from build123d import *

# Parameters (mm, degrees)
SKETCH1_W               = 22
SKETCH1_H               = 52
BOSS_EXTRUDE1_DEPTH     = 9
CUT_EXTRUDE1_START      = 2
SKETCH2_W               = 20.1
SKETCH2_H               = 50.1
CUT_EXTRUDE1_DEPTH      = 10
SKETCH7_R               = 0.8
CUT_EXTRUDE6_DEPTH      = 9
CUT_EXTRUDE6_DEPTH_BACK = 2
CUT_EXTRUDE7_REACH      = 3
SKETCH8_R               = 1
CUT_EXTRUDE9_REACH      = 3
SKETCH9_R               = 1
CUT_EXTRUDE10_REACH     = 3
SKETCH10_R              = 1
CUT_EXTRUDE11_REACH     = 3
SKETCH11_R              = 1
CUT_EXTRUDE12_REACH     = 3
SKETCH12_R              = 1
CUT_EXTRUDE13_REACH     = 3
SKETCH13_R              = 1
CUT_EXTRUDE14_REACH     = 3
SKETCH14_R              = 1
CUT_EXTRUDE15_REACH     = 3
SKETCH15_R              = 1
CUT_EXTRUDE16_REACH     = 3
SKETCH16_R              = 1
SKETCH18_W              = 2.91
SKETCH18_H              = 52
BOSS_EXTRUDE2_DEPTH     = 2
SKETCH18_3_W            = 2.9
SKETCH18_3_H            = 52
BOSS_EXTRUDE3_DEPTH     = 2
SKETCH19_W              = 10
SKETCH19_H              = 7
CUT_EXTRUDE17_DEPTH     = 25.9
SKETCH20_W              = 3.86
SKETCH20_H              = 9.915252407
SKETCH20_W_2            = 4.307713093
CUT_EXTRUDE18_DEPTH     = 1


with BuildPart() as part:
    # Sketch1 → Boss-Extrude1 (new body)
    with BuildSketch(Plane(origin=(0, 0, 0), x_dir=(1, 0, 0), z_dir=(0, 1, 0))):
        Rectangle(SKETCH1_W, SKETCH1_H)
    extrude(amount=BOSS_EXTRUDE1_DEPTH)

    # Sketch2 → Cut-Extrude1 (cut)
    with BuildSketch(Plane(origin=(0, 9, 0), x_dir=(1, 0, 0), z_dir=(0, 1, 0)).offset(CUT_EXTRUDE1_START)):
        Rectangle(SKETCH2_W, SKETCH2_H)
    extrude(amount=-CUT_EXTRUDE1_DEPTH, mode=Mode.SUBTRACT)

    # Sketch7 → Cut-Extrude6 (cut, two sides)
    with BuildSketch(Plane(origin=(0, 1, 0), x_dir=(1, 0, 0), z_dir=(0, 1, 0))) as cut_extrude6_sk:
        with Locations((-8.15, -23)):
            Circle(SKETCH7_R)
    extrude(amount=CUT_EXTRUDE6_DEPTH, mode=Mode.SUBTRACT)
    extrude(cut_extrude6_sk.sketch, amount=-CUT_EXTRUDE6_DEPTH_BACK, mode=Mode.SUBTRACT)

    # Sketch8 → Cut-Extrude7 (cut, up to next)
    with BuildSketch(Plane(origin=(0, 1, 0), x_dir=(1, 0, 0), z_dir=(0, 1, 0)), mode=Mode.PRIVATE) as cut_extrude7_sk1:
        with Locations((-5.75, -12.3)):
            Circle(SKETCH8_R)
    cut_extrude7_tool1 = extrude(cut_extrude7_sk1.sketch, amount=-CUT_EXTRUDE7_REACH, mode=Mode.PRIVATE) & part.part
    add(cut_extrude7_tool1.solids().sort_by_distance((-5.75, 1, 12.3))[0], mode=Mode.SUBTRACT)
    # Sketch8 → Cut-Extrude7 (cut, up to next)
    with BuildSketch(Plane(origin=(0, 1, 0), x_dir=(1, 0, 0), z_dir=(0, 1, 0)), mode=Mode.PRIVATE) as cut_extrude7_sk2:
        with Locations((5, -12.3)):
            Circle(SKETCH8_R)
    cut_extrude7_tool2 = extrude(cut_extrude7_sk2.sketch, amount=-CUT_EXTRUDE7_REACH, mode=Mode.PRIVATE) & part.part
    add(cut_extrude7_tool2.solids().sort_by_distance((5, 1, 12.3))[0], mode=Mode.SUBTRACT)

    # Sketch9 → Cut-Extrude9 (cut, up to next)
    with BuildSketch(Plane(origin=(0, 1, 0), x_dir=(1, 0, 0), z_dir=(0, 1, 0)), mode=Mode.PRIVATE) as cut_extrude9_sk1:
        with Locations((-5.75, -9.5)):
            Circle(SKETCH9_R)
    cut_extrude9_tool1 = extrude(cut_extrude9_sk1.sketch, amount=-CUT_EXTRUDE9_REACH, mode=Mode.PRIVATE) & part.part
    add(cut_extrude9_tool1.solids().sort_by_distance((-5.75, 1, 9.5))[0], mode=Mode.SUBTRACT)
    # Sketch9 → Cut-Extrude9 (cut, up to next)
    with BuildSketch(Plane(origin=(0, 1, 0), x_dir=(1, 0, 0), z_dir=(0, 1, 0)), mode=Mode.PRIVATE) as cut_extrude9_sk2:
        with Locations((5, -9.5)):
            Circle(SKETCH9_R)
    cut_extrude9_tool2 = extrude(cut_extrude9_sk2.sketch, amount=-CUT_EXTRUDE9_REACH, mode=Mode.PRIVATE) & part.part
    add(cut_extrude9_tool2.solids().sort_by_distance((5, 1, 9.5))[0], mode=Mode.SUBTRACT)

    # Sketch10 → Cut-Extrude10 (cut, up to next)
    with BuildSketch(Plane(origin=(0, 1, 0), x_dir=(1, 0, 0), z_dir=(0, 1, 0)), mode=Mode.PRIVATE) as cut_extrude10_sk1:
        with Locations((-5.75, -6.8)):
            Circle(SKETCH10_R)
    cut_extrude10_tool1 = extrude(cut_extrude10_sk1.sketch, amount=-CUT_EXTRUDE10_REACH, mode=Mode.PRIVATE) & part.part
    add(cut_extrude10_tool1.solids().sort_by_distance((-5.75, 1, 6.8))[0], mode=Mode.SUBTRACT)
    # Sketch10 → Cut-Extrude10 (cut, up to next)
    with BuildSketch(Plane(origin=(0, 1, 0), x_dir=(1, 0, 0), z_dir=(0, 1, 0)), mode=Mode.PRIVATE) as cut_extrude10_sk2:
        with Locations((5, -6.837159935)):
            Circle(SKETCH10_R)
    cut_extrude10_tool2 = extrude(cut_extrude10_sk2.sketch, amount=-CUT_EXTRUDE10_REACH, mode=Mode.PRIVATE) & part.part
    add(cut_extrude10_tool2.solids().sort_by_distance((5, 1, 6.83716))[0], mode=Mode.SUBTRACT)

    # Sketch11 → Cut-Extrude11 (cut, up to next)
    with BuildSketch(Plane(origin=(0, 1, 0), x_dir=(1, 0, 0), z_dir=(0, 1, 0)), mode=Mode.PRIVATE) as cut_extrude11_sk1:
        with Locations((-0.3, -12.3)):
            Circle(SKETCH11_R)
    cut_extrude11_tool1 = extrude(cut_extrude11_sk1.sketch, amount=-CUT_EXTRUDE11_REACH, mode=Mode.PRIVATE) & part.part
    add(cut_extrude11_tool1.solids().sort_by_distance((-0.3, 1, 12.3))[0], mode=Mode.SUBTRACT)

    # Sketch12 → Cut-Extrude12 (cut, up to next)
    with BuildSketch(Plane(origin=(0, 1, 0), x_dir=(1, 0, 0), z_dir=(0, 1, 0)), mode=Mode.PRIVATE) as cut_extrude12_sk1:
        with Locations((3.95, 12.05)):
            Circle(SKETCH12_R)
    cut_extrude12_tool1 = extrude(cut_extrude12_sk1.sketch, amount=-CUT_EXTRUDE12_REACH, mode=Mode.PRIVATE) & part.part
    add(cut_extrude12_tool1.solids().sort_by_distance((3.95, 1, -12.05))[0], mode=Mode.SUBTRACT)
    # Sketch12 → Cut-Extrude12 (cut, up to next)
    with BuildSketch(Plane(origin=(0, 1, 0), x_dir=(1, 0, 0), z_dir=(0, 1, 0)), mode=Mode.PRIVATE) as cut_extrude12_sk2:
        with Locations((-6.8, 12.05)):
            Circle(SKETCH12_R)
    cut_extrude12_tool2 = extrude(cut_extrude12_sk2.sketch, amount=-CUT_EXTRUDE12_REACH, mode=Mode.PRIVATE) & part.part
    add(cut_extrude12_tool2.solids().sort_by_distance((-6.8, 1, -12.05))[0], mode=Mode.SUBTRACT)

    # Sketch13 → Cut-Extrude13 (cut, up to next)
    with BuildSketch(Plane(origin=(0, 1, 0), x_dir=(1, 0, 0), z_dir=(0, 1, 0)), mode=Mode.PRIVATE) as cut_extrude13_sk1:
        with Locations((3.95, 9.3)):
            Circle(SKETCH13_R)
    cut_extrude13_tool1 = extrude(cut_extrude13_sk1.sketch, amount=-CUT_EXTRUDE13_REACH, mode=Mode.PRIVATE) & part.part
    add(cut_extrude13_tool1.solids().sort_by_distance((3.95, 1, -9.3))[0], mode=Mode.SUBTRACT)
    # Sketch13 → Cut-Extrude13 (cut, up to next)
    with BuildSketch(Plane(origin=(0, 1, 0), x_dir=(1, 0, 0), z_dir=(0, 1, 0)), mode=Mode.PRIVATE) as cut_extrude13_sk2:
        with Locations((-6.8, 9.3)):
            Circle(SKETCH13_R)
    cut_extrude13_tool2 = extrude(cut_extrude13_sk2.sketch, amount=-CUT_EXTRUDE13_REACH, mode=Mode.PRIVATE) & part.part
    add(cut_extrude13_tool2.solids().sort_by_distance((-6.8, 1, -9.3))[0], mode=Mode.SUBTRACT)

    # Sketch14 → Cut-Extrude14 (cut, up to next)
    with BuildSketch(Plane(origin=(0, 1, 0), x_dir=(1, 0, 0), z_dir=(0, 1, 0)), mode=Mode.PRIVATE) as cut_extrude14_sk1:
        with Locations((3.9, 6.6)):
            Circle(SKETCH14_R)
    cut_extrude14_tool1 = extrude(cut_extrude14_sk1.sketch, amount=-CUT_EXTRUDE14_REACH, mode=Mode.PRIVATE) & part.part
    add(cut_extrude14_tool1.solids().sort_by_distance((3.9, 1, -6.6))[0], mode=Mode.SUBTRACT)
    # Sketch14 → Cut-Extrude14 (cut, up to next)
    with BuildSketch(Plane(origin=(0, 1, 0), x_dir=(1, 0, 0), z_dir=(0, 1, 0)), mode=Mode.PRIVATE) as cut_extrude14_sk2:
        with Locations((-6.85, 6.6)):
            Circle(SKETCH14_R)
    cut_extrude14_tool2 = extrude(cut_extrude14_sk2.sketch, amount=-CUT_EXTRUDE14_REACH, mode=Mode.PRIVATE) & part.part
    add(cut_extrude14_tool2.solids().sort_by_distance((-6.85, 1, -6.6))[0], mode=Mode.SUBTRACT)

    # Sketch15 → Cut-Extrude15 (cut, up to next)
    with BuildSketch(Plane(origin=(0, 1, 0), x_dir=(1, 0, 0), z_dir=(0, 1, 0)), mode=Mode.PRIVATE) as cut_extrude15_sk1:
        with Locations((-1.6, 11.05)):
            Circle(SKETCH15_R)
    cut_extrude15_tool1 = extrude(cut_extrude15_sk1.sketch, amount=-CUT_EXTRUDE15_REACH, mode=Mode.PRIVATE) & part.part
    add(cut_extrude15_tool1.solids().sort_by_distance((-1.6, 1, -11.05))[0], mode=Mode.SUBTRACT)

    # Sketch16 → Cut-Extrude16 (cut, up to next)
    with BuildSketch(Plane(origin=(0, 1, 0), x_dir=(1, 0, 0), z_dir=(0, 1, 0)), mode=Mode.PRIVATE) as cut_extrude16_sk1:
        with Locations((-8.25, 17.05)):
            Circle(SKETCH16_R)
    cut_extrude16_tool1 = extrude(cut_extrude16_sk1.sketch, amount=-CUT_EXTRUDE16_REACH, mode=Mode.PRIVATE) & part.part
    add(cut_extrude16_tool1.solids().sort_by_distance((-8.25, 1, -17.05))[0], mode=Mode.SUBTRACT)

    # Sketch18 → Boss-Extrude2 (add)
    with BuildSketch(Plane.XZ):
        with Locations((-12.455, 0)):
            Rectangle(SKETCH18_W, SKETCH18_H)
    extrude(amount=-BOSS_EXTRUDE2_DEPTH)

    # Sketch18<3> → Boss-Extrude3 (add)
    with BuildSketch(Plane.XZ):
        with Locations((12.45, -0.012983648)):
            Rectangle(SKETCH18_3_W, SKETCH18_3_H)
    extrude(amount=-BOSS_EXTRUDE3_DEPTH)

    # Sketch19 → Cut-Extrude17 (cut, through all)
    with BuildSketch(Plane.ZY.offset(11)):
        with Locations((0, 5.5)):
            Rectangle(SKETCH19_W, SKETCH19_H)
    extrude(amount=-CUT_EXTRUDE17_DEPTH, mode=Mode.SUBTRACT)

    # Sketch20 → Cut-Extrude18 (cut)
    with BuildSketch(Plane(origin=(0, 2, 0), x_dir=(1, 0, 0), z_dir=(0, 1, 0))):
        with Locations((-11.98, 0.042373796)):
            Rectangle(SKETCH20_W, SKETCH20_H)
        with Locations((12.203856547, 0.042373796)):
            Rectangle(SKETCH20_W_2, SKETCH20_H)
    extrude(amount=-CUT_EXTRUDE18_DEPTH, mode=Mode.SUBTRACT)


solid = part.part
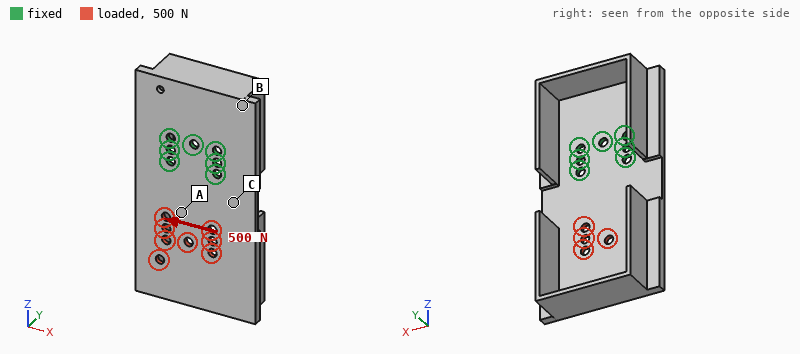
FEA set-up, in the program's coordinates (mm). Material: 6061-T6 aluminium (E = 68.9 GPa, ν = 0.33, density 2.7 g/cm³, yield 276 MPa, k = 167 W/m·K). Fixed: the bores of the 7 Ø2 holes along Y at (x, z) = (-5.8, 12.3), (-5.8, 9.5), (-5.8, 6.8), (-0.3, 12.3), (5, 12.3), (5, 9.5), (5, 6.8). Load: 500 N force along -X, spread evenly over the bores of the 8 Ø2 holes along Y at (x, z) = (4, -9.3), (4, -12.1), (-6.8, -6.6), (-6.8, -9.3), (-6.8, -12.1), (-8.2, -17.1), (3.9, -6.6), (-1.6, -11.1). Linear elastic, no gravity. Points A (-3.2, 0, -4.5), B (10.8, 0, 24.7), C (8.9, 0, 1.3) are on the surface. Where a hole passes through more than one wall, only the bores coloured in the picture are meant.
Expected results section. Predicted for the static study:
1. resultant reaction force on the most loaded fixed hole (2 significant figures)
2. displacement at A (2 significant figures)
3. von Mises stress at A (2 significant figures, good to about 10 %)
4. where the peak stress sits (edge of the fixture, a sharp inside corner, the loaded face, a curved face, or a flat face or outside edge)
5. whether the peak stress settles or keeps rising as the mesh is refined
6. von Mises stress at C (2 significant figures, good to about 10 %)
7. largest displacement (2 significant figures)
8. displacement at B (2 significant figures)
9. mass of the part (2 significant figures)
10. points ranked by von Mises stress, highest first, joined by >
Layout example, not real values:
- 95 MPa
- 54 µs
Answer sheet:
- 460 N
- 20 µm
- 43 MPa
- edge of the fixture
- keeps rising
- 29 MPa
- 57 µm
- 8.7 µm
- 7.0 g
- A > C > B
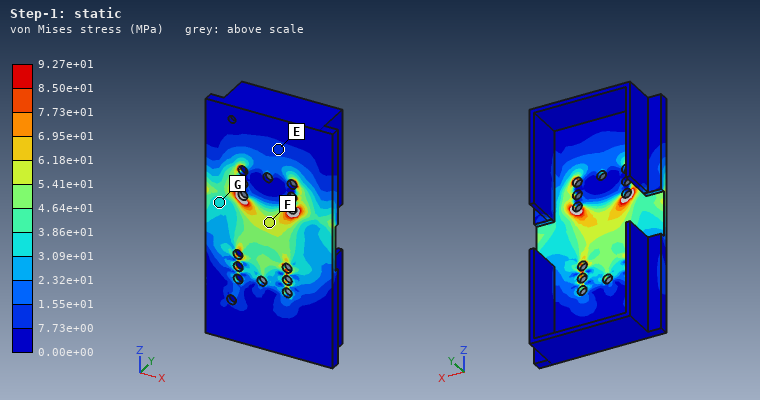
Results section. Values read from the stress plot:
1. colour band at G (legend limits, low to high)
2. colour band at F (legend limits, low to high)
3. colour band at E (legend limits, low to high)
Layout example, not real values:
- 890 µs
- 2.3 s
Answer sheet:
- 3.09e+01 to 3.86e+01 MPa
- 5.41e+01 to 6.18e+01 MPa
- 7.73e+00 to 1.55e+01 MPa
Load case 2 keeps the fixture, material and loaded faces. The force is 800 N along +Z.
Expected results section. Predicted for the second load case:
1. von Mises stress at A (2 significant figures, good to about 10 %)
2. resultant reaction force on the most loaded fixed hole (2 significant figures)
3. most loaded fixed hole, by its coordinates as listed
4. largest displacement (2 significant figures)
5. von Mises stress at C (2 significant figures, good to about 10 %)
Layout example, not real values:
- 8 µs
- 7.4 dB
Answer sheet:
- 39 MPa
- 300 N
- (-5.8, 6.8)
- 20 µm
- 17 MPa
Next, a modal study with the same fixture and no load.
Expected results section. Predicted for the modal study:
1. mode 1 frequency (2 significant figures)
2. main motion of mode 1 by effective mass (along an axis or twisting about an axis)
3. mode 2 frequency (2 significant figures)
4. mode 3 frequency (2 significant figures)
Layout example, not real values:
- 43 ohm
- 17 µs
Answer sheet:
- 550 Hz
- along Y
- 1600 Hz
- 4000 Hz
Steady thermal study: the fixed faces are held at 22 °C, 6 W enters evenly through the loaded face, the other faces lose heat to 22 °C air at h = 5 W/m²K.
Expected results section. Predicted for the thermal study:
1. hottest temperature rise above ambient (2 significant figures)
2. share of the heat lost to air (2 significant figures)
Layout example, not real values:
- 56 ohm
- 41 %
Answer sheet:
- 24 K
- 4.4 %
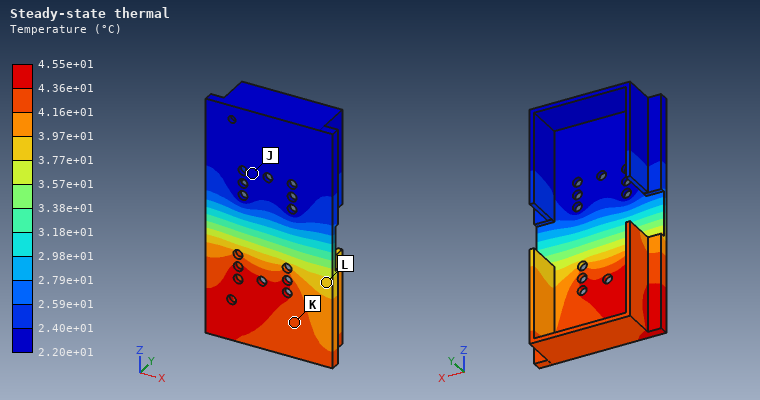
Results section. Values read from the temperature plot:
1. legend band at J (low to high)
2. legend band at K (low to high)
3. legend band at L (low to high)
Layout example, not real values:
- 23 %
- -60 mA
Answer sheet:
- 2.20e+01 to 2.40e+01 °C
- 4.16e+01 to 4.36e+01 °C
- 3.77e+01 to 3.97e+01 °C
